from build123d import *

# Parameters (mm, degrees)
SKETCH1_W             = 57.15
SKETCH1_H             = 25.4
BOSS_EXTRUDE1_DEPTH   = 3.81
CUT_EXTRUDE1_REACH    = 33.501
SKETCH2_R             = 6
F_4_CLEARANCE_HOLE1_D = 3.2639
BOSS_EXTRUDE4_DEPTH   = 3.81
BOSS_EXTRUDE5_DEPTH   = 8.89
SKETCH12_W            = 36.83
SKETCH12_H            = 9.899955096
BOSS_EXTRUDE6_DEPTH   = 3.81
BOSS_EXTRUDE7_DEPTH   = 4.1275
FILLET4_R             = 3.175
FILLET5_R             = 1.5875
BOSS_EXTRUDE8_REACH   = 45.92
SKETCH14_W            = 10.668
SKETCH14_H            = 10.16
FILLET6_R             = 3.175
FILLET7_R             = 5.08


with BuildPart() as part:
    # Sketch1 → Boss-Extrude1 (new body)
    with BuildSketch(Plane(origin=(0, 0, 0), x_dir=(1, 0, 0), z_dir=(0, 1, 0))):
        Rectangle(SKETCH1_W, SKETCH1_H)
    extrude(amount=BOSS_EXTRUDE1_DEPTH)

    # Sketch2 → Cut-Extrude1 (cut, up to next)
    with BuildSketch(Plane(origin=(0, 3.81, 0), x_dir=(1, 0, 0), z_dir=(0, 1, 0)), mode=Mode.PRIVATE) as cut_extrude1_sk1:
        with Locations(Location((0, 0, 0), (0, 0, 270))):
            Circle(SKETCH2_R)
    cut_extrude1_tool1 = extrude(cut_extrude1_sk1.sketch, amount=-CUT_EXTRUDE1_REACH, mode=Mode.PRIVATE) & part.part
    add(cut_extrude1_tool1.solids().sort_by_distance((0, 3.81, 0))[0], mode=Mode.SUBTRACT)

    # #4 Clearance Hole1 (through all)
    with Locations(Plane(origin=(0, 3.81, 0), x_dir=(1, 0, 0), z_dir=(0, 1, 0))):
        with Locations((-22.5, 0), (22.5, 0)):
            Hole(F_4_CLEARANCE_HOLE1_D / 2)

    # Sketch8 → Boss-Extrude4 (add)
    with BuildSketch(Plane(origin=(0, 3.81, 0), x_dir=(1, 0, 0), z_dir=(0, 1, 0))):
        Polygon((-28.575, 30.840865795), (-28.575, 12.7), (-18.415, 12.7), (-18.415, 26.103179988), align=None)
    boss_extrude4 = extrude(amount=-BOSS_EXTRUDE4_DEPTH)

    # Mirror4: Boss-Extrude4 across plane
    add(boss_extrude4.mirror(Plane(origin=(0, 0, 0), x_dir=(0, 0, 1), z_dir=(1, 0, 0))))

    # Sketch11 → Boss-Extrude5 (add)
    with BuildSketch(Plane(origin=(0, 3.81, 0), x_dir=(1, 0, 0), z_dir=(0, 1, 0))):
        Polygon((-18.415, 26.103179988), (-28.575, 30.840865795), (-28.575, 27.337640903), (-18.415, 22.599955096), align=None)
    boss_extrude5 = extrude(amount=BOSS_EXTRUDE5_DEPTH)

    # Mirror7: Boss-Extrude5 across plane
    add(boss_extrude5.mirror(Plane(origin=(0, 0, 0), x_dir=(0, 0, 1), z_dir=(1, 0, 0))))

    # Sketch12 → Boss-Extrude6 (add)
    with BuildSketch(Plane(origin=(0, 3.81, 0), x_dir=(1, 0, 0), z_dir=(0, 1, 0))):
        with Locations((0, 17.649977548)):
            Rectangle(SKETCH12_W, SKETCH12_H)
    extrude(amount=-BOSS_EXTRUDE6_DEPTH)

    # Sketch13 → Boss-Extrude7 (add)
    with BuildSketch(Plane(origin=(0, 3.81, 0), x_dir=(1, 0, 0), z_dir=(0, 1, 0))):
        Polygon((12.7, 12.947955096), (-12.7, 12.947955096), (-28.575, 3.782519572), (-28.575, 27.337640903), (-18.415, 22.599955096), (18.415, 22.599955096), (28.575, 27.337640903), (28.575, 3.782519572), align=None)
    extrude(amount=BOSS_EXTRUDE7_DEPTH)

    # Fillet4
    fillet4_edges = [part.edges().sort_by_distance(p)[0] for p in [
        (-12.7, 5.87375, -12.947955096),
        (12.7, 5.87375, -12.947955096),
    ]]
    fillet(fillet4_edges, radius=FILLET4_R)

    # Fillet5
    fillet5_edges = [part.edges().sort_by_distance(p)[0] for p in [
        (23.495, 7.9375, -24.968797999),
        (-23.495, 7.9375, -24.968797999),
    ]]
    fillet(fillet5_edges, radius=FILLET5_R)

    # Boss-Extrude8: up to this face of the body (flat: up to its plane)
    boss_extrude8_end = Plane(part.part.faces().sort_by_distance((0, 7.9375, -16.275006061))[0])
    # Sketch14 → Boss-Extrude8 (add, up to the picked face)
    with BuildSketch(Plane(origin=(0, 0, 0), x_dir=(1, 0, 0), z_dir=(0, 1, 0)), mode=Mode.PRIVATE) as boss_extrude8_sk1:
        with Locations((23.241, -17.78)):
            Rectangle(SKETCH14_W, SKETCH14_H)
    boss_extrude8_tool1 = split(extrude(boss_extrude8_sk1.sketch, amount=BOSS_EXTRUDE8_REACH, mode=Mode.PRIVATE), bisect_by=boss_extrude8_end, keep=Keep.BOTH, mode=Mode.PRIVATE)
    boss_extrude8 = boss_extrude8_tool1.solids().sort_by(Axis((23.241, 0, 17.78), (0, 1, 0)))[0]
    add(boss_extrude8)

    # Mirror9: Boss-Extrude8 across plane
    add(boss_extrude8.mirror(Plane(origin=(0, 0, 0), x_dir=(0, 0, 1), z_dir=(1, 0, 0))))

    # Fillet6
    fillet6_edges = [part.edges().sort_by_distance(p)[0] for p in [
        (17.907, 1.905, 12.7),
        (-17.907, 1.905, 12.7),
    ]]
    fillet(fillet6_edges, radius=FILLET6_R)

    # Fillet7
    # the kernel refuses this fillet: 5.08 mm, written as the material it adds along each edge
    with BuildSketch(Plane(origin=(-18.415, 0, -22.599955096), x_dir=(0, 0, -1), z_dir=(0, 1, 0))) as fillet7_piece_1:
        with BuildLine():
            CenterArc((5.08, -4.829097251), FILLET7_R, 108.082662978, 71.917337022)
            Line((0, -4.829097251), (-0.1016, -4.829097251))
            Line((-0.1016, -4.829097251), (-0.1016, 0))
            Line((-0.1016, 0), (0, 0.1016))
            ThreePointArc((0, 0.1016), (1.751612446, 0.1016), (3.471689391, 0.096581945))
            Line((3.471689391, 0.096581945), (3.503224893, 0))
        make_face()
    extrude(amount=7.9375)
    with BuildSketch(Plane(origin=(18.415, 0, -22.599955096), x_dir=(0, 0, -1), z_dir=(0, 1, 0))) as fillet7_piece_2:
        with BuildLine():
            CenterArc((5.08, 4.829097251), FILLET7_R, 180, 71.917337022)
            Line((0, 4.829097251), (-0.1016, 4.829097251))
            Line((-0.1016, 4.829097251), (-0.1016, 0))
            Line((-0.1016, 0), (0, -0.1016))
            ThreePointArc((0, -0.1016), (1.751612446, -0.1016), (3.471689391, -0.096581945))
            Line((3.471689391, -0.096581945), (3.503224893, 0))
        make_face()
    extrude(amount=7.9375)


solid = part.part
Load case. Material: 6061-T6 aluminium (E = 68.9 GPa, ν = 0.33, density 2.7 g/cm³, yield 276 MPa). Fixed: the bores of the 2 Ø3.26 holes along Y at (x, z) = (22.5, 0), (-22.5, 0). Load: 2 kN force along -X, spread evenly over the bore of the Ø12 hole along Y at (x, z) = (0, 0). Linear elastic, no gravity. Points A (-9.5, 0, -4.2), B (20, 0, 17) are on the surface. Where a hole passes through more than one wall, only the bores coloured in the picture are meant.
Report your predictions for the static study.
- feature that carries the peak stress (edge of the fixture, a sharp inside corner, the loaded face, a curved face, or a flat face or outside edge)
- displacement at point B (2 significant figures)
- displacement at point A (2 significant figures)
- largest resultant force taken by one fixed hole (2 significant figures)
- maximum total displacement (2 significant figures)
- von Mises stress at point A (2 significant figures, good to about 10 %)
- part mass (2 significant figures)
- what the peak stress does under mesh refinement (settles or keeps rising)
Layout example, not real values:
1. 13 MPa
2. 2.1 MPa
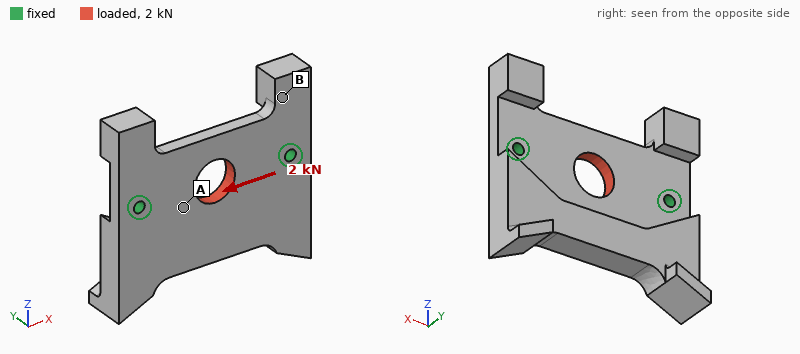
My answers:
1. edge of the fixture
2. 4.2 µm
3. 3.6 µm
4. 1.0 kN
5. 5.7 µm
6. 15 MPa
7. 36 g
8. keeps rising
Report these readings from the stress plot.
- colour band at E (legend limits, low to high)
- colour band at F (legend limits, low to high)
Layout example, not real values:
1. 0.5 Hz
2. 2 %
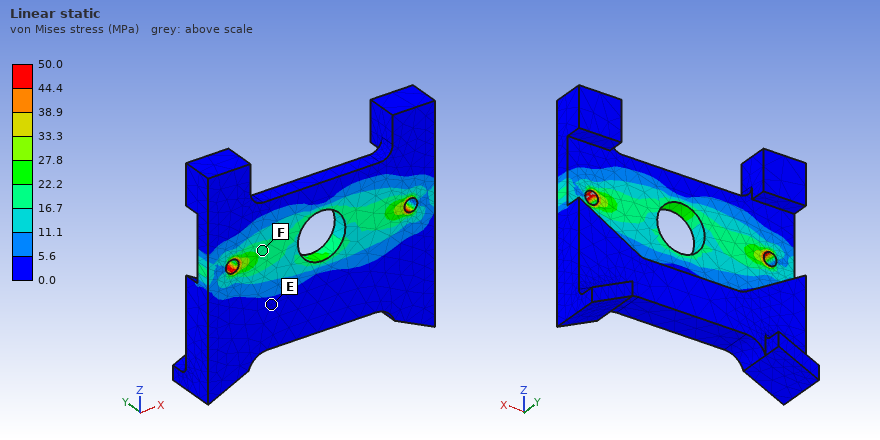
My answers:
1. 0.0 to 5.6 MPa
2. 16.7 to 22.2 MPa
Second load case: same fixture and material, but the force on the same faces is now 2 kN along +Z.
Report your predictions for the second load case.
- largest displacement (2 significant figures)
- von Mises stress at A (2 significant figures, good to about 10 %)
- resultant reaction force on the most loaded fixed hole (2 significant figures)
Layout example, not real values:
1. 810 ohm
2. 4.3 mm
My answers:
1. 14 µm
2. 18 MPa
3. 1.0 kN
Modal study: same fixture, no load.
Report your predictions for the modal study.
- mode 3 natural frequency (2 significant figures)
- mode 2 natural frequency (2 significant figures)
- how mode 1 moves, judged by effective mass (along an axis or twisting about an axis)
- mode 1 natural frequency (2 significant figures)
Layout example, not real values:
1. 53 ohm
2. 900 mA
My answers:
1. 5100 Hz
2. 5100 Hz
3. along Y
4. 2600 Hz
